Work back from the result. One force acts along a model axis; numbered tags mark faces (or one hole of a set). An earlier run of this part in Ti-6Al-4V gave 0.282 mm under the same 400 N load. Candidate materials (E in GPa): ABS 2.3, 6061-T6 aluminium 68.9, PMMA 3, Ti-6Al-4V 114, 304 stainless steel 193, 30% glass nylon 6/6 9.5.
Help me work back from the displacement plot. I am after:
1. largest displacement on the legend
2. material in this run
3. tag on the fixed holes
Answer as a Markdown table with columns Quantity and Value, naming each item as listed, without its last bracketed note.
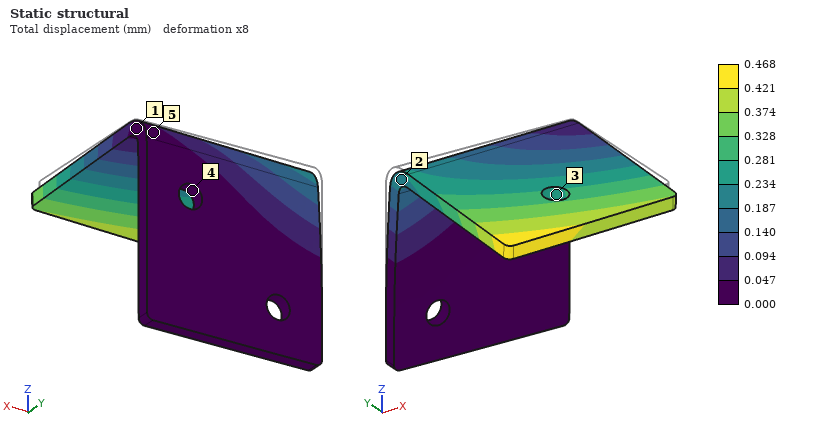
| Quantity | Value |
|---|---|
| largest displacement on the legend | 0.468 mm |
| material in this run | 6061-T6 aluminium |
| tag on the fixed holes | 4 |
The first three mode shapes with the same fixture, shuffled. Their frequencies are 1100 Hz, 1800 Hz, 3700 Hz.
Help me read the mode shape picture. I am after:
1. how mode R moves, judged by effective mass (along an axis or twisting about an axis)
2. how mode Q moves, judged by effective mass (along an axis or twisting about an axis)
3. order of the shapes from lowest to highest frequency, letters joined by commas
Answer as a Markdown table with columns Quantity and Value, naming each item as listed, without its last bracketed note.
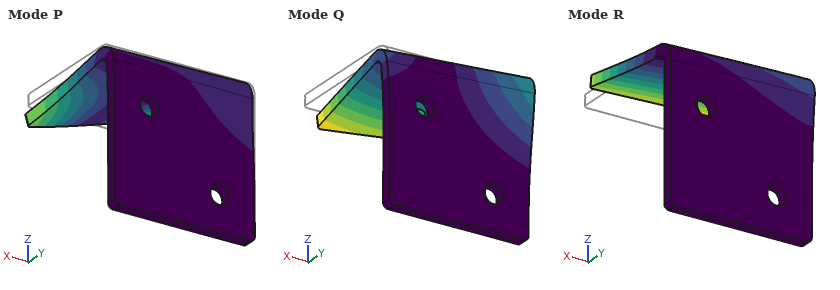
| Quantity | Value |
|---|---|
| how mode R moves, judged by effective mass | along Z |
| how mode Q moves, judged by effective mass | along X |
| order of the shapes from lowest to highest frequency, letters joined by commas | R, Q, P |
